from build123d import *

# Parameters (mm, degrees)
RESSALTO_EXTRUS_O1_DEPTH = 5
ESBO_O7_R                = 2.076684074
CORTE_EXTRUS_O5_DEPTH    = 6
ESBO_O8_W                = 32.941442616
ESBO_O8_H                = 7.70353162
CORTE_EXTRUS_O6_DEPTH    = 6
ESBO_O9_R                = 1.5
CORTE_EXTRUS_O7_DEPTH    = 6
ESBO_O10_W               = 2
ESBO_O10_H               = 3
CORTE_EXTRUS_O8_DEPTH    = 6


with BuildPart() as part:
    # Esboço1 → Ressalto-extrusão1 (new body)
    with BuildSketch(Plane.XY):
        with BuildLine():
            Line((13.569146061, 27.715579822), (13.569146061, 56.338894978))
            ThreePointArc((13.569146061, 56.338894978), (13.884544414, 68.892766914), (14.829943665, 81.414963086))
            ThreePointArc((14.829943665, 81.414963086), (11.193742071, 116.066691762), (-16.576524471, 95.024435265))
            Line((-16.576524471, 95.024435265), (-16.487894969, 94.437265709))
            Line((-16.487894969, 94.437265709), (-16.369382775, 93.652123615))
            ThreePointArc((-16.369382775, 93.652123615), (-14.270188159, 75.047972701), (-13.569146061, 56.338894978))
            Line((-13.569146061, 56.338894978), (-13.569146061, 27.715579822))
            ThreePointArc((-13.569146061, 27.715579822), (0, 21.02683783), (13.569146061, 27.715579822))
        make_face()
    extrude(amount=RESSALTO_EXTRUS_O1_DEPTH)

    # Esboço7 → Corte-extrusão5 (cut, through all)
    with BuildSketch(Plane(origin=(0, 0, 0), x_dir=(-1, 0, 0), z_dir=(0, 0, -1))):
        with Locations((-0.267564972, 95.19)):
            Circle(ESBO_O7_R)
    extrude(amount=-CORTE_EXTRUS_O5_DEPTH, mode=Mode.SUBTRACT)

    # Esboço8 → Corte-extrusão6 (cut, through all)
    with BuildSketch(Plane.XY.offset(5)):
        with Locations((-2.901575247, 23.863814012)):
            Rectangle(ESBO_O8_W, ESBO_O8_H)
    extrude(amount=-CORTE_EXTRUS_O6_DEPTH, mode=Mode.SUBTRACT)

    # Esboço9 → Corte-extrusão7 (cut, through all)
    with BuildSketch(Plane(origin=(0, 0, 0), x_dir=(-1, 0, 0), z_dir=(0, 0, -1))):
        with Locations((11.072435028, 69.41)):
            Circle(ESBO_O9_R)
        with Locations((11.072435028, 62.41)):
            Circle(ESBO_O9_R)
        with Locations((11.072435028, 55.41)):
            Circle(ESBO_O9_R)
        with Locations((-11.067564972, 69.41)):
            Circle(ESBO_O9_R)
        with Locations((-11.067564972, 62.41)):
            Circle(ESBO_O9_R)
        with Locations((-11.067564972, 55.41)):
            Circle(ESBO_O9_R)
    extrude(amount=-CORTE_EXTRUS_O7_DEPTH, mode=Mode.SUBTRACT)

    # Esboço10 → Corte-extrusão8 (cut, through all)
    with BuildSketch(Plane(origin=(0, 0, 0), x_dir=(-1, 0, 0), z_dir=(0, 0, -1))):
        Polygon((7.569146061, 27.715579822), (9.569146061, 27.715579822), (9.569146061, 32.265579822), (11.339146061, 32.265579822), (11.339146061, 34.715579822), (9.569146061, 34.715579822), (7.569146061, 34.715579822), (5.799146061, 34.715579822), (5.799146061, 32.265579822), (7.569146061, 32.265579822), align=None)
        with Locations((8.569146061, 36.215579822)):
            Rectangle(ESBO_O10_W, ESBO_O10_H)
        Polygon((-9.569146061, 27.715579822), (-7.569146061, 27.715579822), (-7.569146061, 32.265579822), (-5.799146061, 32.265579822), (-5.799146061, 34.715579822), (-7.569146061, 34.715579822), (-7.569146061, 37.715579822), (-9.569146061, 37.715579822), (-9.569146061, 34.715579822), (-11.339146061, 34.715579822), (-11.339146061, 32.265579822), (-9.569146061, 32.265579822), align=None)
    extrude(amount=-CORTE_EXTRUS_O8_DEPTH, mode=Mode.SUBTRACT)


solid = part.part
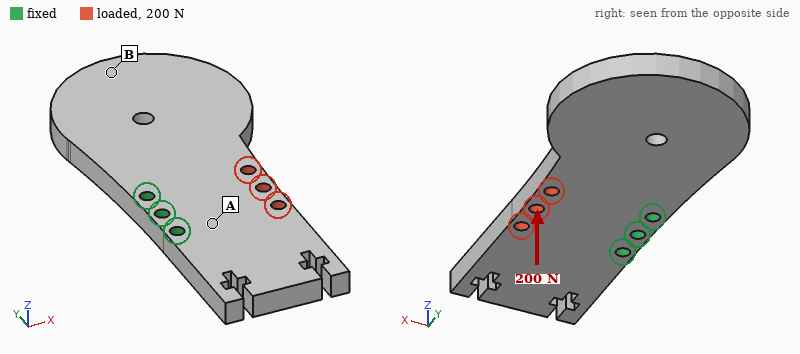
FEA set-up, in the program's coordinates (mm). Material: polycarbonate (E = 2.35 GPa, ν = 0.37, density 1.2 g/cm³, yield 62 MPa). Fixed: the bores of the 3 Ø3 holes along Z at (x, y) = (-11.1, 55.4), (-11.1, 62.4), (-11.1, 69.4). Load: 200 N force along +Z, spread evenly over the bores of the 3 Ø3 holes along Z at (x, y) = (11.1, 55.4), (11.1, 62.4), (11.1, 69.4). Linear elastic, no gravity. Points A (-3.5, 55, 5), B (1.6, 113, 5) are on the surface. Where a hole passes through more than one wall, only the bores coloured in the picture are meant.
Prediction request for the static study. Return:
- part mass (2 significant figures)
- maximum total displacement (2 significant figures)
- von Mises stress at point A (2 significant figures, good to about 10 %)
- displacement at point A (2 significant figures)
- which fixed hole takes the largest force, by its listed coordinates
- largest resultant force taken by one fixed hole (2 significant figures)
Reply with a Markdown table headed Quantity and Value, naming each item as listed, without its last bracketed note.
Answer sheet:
| Quantity | Value |
|---|---|
| part mass | 16 g |
| maximum total displacement | 1.0 mm |
| von Mises stress at point A | 17 MPa |
| displacement at point A | 0.18 mm |
| which fixed hole takes the largest force, by its listed coordinates | (-11.1, 62.4) |
| largest resultant force taken by one fixed hole | 93 N |
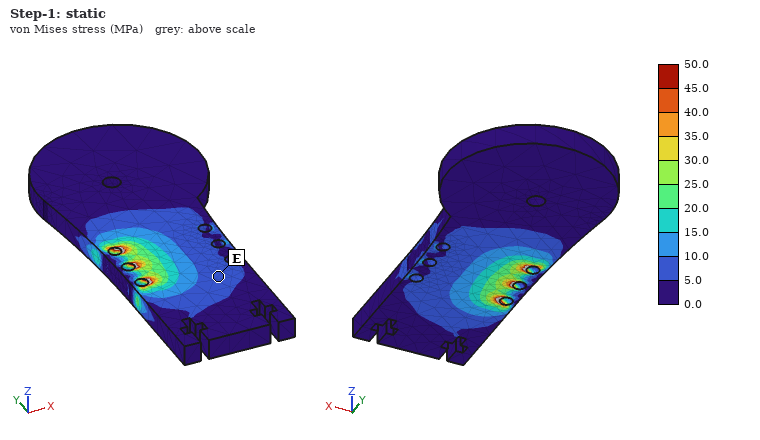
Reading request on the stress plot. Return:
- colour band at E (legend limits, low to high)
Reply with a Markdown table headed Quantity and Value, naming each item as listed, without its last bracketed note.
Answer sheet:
| Quantity | Value |
|---|---|
| colour band at E | 5.0 to 10.0 MPa |
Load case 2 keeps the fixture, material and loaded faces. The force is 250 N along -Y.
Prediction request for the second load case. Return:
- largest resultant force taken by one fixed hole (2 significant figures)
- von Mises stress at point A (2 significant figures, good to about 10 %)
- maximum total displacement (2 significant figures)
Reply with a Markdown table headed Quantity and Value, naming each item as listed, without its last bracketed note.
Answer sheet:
| Quantity | Value |
|---|---|
| largest resultant force taken by one fixed hole | 330 N |
| von Mises stress at point A | 5.6 MPa |
| maximum total displacement | 0.32 mm |
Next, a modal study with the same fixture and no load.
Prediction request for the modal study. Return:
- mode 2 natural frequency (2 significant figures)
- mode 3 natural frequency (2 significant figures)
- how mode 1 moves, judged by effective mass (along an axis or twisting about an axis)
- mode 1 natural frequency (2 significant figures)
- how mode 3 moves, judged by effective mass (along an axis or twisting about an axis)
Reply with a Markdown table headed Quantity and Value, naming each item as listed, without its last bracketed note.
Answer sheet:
| Quantity | Value |
|---|---|
| mode 2 natural frequency | 980 Hz |
| mode 3 natural frequency | 1100 Hz |
| how mode 1 moves, judged by effective mass | along Z |
| mode 1 natural frequency | 380 Hz |
| how mode 3 moves, judged by effective mass | along Z |
